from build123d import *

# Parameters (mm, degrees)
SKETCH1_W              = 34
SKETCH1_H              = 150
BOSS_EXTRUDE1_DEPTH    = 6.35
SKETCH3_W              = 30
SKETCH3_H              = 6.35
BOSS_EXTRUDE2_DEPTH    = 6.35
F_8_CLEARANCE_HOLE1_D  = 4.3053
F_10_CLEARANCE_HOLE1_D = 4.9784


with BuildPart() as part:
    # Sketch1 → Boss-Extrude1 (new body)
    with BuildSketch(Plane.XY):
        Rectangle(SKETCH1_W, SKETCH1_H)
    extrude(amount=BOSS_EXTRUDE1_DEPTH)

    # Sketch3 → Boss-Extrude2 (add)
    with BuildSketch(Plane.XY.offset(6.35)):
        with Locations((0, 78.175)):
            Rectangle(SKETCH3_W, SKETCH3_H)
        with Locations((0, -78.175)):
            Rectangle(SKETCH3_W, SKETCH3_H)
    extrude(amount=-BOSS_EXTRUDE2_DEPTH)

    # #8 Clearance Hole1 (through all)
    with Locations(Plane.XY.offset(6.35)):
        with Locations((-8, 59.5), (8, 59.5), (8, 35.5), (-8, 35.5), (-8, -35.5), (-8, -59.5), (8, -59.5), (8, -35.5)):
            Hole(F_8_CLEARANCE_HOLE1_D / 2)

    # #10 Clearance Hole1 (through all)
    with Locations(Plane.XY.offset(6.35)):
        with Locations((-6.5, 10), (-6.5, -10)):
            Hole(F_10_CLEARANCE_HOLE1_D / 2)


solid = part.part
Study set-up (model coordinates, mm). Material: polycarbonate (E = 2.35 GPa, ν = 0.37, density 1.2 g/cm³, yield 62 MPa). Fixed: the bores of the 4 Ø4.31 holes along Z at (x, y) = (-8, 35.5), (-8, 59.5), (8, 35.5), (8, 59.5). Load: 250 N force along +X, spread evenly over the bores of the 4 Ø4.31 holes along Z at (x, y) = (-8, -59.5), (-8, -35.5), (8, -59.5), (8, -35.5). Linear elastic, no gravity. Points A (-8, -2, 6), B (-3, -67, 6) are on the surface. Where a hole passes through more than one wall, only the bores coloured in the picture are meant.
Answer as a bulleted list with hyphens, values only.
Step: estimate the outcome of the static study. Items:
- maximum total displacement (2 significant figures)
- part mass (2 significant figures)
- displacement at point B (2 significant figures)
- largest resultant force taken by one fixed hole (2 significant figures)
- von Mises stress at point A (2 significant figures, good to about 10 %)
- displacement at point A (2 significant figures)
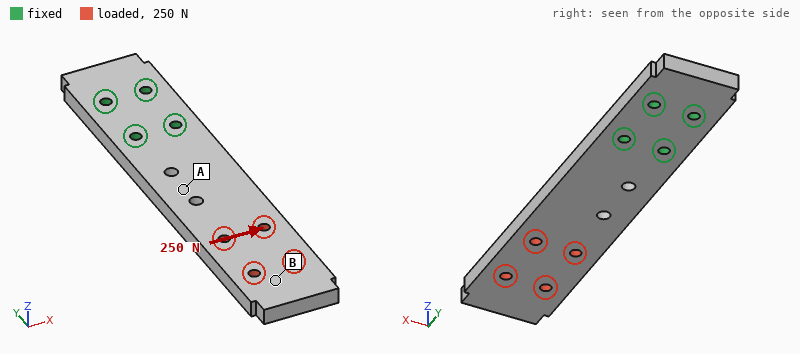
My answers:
- 2.0 mm
- 41 g
- 1.7 mm
- 860 N
- 4.2 MPa
- 0.39 mm
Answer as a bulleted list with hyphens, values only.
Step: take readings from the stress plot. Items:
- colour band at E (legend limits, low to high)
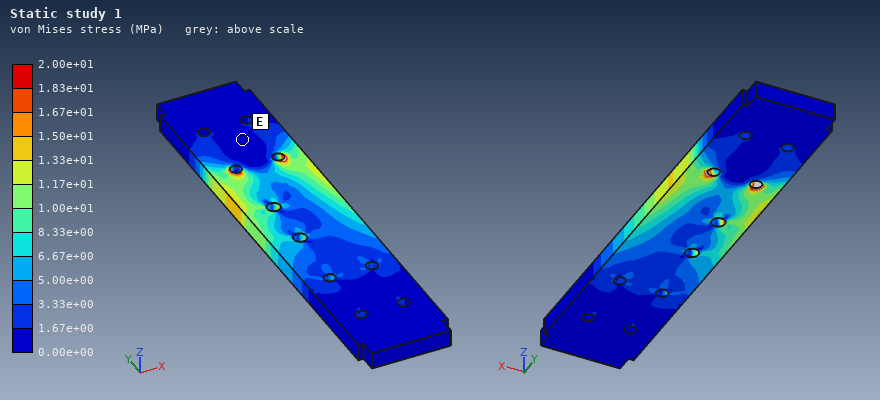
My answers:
- 0.00e+00 to 1.67e+00 MPa
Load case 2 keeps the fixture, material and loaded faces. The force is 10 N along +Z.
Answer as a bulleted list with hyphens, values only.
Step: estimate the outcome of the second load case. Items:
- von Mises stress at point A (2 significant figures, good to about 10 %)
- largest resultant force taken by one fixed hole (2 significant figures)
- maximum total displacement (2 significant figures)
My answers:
- 1.7 MPa
- 8.3 N
- 1.8 mm
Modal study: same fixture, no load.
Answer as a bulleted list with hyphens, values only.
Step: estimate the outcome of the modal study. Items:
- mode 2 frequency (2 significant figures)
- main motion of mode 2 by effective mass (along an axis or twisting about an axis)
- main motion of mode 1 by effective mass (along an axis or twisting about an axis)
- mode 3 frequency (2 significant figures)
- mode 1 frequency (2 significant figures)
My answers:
- 500 Hz
- along X
- along Z
- 650 Hz
- 110 Hz
